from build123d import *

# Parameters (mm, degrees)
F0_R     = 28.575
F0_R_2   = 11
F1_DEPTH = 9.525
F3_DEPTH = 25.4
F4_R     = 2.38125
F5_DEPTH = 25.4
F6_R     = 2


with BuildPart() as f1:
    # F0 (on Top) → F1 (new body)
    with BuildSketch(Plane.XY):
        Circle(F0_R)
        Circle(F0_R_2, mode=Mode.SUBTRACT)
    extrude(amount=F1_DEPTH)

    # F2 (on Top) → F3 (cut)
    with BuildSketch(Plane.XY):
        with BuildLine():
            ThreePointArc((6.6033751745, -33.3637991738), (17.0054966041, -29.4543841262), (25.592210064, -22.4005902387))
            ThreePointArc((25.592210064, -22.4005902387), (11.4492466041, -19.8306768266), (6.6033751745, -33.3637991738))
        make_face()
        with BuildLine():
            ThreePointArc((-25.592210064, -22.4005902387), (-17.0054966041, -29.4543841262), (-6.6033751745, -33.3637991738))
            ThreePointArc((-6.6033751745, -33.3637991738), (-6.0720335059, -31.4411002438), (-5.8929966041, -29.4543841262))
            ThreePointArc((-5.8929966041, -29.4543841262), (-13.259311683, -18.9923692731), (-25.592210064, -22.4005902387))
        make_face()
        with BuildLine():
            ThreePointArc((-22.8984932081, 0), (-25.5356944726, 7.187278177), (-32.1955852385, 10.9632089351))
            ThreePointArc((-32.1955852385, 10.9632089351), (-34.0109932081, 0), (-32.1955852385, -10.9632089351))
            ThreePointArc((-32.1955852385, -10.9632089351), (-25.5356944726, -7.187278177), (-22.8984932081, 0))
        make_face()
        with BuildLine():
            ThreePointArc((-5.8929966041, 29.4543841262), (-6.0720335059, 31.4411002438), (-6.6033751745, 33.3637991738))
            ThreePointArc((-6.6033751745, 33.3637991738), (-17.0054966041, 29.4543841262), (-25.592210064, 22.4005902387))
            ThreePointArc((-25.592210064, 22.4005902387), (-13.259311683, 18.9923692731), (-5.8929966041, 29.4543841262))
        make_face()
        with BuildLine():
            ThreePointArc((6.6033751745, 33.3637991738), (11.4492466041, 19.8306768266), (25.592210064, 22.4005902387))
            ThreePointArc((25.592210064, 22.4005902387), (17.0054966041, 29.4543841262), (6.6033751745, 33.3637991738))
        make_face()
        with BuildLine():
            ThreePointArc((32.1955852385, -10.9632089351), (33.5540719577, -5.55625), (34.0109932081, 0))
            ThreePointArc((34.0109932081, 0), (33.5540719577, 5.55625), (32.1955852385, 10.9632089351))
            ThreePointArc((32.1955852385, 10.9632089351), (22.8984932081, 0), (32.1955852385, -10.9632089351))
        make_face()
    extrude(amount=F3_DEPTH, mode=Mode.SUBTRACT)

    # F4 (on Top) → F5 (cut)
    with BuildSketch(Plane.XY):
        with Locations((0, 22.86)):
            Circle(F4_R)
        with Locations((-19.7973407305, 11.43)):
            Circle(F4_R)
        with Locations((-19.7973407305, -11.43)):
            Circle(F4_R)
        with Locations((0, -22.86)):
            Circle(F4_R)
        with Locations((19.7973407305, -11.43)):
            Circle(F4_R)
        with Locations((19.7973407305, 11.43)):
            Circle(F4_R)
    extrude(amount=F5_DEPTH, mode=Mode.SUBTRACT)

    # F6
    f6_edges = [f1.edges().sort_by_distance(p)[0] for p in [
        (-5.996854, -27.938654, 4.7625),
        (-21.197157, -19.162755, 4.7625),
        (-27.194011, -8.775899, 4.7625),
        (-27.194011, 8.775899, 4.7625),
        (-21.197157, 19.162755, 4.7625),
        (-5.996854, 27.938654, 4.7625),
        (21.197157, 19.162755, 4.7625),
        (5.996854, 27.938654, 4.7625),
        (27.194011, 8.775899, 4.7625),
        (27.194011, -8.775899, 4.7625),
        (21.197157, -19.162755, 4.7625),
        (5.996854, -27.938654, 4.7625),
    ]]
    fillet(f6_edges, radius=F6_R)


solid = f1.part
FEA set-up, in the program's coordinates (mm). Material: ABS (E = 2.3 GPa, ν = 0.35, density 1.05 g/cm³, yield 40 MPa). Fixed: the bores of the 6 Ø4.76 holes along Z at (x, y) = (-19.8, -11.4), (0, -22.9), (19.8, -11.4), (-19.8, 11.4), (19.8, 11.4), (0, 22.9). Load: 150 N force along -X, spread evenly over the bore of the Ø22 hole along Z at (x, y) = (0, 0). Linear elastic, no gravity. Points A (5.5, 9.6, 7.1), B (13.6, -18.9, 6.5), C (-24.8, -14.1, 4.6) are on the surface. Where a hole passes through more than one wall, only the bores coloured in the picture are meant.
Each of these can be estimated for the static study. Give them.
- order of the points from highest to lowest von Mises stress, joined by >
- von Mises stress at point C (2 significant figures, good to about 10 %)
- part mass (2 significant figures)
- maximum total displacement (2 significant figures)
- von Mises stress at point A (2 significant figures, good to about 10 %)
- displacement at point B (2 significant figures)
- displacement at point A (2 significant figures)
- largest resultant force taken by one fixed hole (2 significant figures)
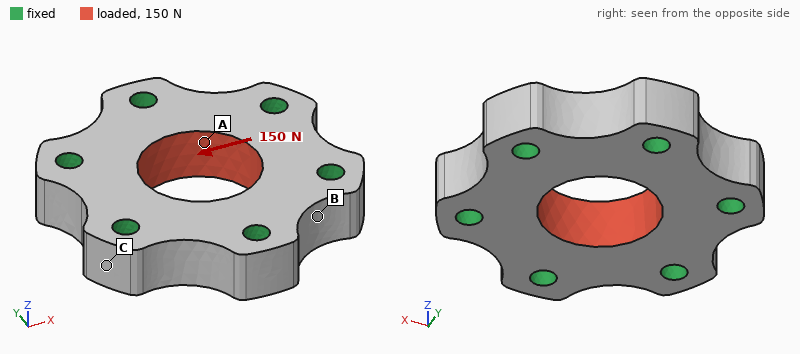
A > C > B
0.15 MPa
17 g
1.8 µm
0.36 MPa
0.63 µm
1.6 µm
34 N
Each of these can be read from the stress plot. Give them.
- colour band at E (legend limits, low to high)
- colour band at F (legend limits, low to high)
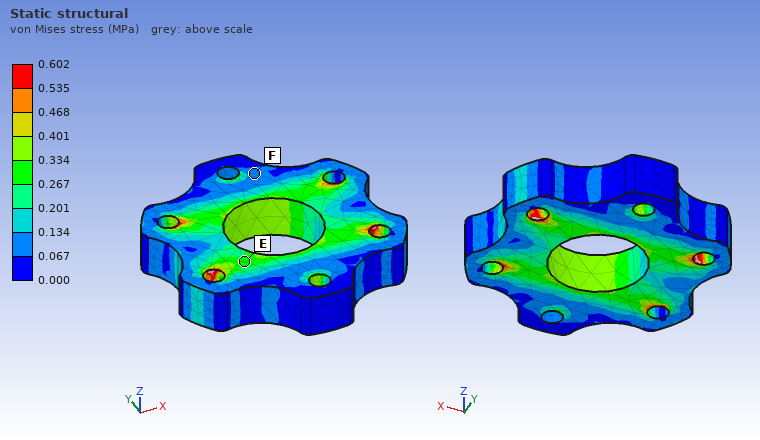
0.267 to 0.334 MPa
0.067 to 0.134 MPa
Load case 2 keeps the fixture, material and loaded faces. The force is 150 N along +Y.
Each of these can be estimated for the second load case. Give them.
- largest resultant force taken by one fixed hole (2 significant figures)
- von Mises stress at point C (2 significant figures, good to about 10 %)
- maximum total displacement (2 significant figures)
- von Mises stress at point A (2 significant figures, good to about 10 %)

39 N
0.084 MPa
1.8 µm
0.26 MPa
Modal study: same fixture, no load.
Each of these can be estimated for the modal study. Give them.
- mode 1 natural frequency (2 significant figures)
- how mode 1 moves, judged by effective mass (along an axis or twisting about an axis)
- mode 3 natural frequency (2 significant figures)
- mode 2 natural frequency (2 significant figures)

12 kHz
along Z
14 kHz
14 kHz
